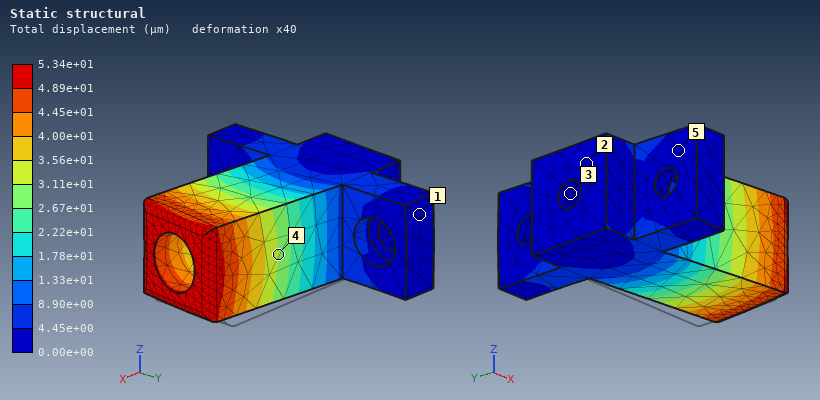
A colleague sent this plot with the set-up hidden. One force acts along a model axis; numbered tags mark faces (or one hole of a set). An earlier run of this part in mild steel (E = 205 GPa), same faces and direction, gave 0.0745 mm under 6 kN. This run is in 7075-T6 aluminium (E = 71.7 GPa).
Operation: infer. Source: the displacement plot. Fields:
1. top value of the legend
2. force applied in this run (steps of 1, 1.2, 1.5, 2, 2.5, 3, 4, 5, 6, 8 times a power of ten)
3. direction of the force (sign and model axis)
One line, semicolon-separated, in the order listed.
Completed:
5.34e+01 µm; 1.5 kN; -Y
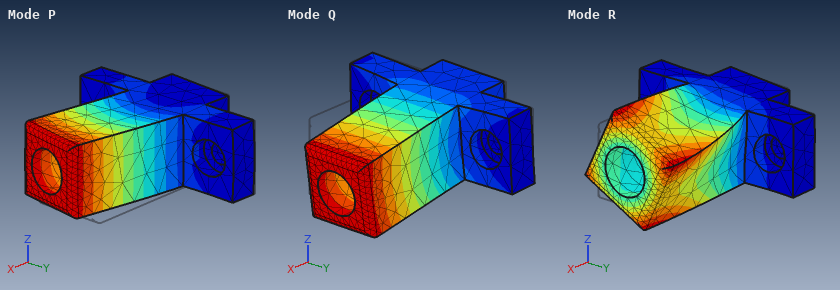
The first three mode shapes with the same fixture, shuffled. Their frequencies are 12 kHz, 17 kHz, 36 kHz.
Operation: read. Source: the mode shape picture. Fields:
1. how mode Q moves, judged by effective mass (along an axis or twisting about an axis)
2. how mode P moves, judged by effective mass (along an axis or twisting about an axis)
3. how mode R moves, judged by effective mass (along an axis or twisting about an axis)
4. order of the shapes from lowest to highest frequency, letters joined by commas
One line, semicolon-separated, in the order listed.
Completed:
along Z; along Y; twisting about X; Q, P, R
